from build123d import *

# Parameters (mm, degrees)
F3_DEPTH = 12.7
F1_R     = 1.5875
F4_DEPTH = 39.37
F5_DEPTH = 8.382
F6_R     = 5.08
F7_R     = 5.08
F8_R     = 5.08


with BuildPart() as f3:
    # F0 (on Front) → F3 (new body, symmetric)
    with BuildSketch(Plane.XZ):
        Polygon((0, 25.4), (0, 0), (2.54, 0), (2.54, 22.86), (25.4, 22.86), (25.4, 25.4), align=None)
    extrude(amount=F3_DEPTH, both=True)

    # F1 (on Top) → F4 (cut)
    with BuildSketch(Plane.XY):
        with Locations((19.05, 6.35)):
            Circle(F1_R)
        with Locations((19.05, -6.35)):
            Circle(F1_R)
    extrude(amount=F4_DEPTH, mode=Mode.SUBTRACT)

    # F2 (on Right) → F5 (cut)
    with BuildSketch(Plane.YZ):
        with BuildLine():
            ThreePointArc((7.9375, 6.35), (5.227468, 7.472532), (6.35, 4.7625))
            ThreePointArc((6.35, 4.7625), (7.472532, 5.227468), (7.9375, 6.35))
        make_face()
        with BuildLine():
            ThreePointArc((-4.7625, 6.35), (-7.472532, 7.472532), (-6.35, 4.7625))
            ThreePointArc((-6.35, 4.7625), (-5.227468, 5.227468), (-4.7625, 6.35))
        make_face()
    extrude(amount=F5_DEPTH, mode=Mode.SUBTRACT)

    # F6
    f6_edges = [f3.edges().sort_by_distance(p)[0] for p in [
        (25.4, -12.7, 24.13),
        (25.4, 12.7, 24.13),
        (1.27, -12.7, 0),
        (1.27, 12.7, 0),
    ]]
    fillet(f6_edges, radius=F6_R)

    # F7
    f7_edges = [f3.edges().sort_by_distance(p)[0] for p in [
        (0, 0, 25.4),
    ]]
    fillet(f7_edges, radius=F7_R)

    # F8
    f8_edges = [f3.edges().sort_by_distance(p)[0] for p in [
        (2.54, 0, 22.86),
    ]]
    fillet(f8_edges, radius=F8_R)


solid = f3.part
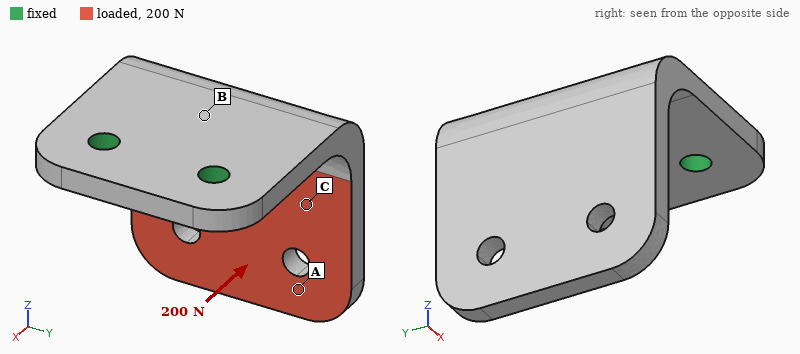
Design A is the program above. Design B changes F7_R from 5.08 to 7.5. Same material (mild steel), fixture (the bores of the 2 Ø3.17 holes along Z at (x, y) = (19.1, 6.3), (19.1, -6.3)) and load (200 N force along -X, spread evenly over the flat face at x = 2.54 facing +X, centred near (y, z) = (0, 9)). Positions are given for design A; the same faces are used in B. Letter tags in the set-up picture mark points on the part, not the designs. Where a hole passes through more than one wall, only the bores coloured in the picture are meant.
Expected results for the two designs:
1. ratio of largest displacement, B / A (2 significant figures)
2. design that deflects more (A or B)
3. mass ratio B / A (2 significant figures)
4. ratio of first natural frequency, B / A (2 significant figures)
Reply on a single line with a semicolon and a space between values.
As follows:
1.1; B; 0.94; 0.98
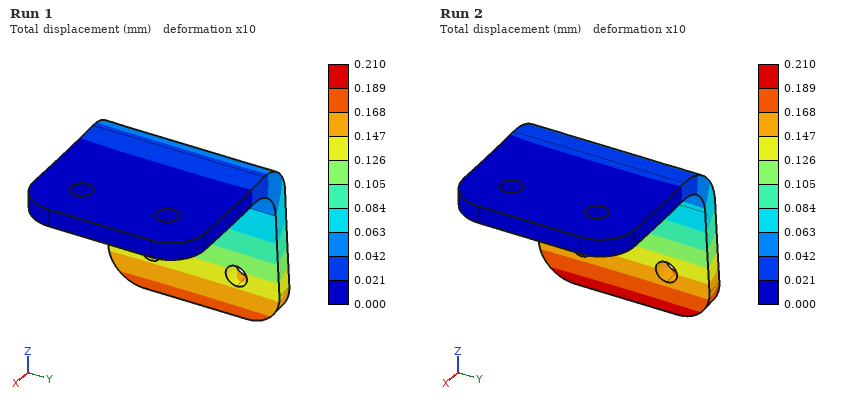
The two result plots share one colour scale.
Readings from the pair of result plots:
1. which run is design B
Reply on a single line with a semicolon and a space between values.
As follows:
Run 2
